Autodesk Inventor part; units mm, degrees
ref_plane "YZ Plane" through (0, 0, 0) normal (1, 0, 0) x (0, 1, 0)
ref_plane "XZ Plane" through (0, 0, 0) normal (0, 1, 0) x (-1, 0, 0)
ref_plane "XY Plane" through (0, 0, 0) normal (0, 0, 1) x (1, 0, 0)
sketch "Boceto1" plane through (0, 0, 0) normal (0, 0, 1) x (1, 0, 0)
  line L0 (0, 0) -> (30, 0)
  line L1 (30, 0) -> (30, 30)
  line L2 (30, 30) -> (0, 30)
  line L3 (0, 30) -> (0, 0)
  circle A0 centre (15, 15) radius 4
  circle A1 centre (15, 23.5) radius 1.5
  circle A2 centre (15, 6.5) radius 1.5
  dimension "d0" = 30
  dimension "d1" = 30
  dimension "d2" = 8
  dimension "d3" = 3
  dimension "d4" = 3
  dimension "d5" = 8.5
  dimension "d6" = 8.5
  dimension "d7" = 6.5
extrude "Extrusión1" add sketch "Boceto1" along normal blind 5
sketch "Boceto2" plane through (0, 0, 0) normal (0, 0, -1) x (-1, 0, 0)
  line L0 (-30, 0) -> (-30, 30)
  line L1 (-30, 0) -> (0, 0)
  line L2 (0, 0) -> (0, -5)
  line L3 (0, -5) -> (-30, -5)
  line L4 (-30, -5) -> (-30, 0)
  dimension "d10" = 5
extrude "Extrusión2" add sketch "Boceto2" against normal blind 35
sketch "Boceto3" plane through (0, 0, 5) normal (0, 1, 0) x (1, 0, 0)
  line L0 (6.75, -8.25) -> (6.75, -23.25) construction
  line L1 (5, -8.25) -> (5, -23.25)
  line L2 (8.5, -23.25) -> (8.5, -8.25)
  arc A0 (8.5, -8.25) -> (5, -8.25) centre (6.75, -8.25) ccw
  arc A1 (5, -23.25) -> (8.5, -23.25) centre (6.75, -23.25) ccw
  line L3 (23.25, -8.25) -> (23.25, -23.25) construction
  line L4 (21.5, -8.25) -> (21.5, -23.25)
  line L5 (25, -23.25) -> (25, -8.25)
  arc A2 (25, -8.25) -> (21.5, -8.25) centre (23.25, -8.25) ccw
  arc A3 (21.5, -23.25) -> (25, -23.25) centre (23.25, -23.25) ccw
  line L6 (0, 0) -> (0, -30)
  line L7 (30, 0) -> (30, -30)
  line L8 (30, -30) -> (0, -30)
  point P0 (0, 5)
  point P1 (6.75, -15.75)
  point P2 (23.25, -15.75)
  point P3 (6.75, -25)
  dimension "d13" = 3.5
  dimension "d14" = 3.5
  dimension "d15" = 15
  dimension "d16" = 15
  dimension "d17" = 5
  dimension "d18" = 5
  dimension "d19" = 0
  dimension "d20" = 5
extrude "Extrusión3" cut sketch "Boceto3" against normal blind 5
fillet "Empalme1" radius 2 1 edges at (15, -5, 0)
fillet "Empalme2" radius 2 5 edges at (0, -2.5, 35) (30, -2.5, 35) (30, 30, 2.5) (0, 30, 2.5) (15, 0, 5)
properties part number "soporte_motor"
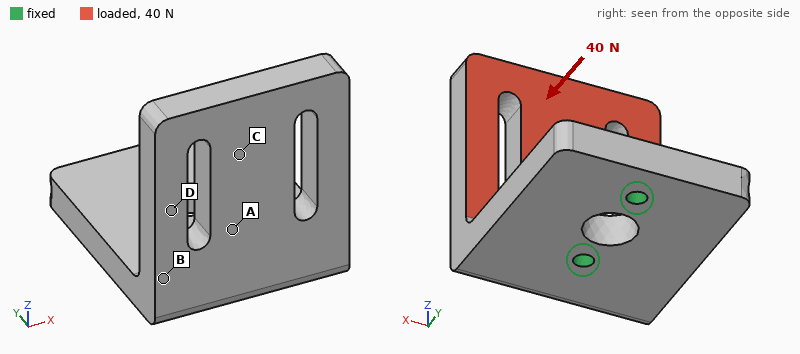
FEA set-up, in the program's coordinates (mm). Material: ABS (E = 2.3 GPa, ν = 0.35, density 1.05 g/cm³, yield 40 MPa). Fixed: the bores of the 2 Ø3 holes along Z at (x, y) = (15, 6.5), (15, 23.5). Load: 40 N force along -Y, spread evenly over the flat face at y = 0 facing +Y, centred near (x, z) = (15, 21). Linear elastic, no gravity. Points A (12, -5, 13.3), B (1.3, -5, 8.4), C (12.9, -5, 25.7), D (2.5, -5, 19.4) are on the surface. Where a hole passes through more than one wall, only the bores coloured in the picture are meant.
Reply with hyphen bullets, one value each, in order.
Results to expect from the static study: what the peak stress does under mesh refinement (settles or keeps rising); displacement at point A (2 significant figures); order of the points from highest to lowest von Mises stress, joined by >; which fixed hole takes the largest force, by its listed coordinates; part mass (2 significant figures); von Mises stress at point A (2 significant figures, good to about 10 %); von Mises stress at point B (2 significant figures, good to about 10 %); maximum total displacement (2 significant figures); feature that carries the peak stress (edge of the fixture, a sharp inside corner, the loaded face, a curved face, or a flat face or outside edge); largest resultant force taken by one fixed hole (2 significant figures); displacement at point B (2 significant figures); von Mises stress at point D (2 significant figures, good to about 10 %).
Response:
- keeps rising
- 0.17 mm
- B > A > D > C
- (15, 6.5)
- 9.2 g
- 3.1 MPa
- 4.2 MPa
- 0.57 mm
- edge of the fixture
- 39 N
- 0.11 mm
- 1.9 MPa
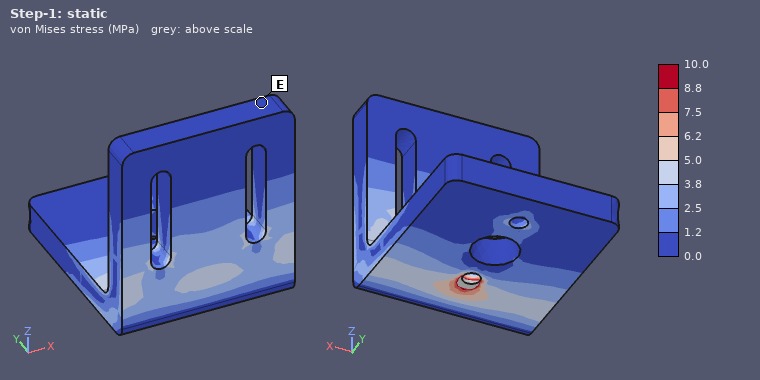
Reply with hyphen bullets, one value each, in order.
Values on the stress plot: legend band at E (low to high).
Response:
- 0.0 to 1.2 MPa
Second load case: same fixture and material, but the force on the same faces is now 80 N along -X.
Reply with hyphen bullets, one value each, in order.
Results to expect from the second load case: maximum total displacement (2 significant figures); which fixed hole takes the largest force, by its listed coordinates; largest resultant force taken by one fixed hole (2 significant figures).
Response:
- 0.61 mm
- (15, 6.5)
- 100 N
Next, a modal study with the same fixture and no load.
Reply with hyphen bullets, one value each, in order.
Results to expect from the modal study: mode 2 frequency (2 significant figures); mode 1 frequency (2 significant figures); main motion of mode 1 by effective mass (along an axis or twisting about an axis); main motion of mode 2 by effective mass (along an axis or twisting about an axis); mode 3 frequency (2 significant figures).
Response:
- 1100 Hz
- 830 Hz
- along Y
- along X
- 2300 Hz
